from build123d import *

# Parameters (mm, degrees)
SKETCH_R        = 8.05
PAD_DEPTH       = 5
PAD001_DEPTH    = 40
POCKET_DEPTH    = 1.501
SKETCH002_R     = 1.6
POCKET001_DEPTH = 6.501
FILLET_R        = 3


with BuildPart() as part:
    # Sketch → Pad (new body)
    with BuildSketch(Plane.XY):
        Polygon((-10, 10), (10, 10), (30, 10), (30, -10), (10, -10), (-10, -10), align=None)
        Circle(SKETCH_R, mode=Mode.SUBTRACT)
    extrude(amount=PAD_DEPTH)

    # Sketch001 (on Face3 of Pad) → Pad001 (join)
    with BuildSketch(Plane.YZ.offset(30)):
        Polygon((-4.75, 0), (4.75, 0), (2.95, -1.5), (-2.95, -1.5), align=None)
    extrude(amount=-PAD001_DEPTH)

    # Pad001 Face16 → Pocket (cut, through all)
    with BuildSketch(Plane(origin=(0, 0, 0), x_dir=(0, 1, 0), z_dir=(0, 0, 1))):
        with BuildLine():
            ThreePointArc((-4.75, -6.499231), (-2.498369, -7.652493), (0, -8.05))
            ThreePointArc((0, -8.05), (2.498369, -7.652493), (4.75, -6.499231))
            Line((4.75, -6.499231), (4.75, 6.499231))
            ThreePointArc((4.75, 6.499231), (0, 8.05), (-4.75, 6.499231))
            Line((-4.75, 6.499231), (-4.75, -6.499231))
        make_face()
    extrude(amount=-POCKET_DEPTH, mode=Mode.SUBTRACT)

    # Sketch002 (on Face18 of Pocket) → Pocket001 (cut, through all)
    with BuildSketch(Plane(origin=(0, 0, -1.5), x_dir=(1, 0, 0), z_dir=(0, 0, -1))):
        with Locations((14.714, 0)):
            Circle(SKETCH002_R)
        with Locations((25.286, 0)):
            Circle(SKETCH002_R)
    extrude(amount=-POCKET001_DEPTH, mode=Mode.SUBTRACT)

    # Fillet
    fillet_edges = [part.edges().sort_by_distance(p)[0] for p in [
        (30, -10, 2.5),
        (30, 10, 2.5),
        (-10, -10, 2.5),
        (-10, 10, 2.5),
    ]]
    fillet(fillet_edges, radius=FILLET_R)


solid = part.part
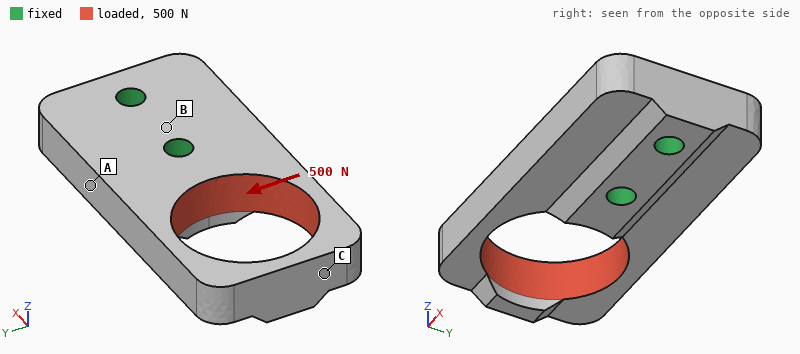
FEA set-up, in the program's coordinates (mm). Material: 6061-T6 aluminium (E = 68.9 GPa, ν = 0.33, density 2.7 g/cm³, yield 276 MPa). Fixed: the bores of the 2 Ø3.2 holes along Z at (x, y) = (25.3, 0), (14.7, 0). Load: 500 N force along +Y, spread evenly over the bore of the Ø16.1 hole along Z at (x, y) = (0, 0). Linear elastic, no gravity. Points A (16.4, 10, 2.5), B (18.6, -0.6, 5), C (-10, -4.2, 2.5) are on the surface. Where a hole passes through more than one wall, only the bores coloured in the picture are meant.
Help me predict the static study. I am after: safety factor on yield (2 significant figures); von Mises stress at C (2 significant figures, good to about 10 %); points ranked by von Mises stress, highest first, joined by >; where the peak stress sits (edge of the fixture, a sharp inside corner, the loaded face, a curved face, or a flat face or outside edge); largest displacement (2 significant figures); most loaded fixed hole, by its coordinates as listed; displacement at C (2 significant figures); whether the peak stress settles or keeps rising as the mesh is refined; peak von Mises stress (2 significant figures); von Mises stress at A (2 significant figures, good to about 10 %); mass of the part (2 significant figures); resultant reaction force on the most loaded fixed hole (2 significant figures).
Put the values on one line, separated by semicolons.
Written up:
3.0; 38 MPa; C > A > B; the loaded face; 68 µm; (14.7, 0); 65 µm; settles; 91 MPa; 20 MPa; 8.4 g; 980 N
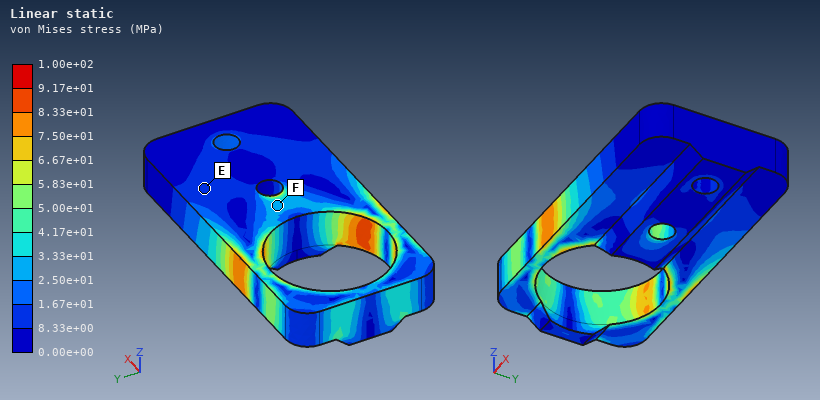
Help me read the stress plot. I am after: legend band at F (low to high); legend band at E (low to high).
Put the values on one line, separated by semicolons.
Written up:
2.50e+01 to 3.33e+01 MPa; 8.33e+00 to 1.67e+01 MPa
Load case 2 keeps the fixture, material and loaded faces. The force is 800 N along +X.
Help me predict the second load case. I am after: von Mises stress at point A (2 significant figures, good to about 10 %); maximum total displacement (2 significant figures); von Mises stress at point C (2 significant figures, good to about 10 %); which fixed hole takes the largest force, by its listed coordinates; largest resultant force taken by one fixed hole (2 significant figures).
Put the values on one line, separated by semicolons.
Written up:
11 MPa; 23 µm; 18 MPa; (14.7, 0); 490 N
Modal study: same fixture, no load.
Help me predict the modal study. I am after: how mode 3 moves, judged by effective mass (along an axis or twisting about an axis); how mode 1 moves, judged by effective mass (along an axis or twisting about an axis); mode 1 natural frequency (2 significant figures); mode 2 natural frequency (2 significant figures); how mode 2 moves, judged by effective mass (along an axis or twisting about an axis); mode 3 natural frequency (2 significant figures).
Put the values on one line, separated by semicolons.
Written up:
twisting about X; along Z; 6100 Hz; 9100 Hz; along Y; 12 kHz
